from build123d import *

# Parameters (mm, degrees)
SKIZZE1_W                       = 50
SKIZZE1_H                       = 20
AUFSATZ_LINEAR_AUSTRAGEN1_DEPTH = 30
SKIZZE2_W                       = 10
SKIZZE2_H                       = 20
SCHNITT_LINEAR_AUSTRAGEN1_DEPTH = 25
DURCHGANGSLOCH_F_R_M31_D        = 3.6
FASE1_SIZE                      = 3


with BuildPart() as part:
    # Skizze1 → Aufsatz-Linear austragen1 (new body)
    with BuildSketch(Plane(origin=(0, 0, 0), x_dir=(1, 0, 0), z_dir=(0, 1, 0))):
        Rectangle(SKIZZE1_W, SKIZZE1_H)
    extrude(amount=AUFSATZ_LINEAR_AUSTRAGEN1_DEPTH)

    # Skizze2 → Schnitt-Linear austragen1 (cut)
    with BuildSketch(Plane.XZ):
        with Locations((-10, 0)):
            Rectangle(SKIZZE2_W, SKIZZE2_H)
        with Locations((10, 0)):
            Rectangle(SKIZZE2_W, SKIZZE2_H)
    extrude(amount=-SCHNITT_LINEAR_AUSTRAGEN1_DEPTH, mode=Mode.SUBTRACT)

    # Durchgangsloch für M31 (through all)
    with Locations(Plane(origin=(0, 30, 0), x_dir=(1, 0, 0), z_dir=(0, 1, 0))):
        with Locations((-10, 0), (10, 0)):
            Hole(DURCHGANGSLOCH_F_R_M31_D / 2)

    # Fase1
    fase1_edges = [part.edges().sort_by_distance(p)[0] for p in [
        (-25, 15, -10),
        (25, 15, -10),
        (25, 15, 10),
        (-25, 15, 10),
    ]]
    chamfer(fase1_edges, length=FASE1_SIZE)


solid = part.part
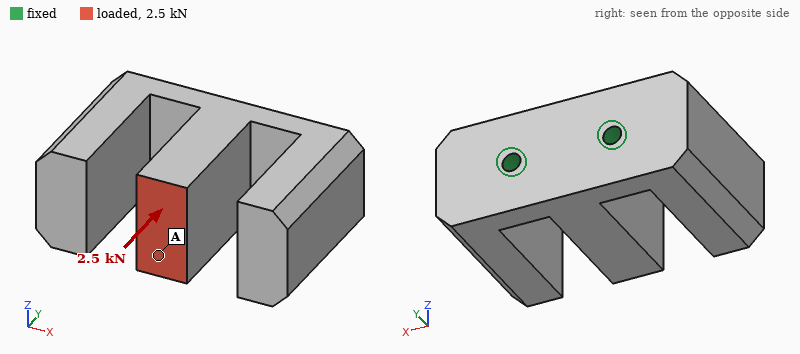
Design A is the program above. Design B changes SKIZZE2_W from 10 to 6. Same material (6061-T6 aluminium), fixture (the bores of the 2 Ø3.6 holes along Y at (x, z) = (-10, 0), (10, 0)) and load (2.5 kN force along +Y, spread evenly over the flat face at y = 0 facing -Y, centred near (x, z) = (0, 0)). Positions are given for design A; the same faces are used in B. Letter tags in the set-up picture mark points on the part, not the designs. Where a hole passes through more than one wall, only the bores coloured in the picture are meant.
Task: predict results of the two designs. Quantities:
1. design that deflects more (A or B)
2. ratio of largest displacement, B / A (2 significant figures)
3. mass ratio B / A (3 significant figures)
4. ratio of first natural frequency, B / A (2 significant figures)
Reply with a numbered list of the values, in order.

1. A
2. 0.66
3. 1.21
4. 1.1
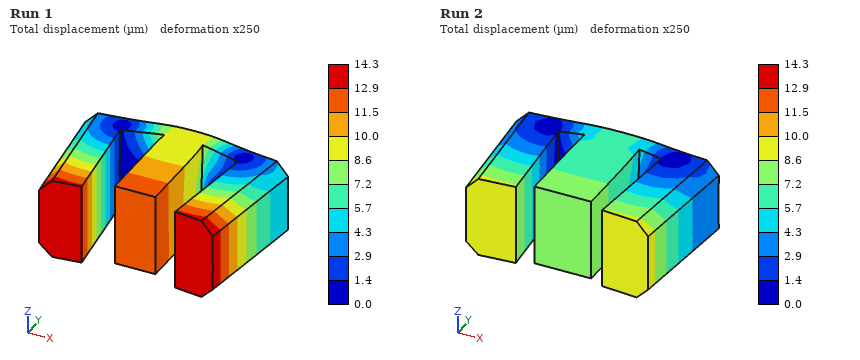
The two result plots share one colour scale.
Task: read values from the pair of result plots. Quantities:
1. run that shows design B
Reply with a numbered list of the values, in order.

1. Run 2
